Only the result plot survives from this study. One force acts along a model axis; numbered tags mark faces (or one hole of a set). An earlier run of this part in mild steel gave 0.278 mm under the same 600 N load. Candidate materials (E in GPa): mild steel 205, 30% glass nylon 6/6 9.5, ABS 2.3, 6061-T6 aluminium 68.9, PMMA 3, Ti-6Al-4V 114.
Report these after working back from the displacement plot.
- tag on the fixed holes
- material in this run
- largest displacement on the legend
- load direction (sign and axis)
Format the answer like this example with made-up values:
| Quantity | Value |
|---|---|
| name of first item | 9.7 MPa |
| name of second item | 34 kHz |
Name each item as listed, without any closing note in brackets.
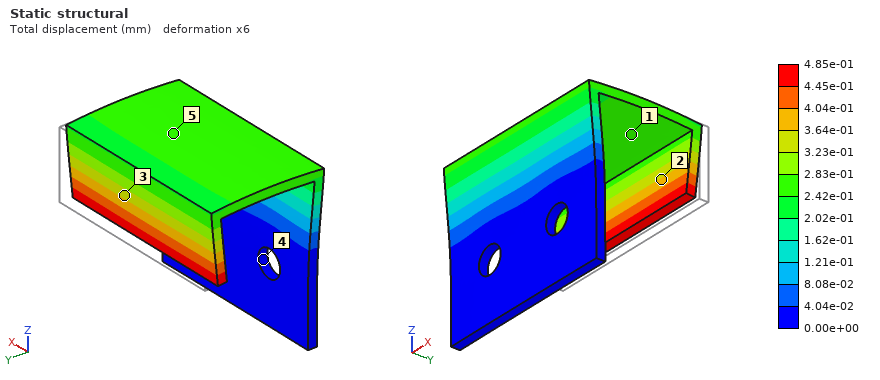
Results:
| Quantity | Value |
|---|---|
| tag on the fixed holes | 4 |
| material in this run | Ti-6Al-4V |
| largest displacement on the legend | 4.85e-01 mm |
| load direction | -Y |
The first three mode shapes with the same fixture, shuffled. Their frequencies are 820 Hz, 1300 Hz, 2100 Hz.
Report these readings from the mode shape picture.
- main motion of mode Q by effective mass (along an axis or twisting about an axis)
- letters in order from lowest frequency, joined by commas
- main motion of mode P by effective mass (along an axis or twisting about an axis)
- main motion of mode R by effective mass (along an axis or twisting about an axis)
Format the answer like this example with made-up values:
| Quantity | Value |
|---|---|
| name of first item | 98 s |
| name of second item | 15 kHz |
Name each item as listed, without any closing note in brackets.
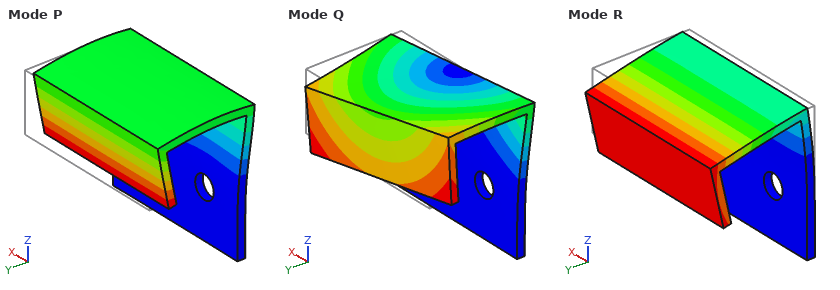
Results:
| Quantity | Value |
|---|---|
| main motion of mode Q by effective mass | along X |
| letters in order from lowest frequency, joined by commas | R, Q, P |
| main motion of mode P by effective mass | along Y |
| main motion of mode R by effective mass | along Z |
